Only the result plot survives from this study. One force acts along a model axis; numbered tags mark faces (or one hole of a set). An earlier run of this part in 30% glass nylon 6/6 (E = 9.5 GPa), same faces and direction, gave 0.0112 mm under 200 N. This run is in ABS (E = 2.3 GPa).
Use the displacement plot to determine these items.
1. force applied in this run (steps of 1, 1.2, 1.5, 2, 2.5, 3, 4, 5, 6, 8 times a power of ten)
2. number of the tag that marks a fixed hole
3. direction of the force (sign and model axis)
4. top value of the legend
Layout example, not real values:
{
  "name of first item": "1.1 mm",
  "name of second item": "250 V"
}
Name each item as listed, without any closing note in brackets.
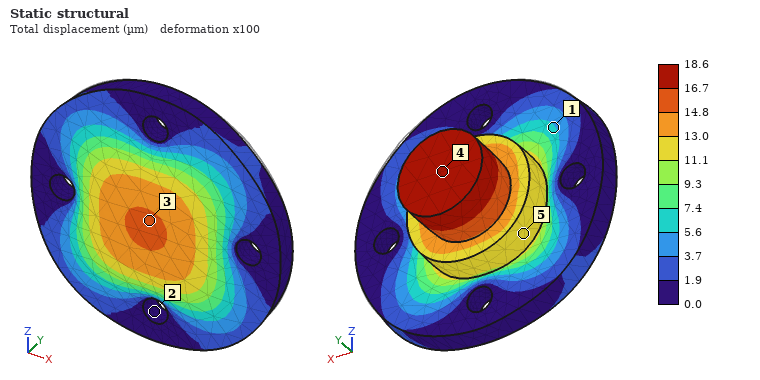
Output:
{
  "force applied in this run": "80 N",
  "number of the tag that marks a fixed hole": "2",
  "direction of the force": "-Y",
  "top value of the legend": "18.6 µm"
}
